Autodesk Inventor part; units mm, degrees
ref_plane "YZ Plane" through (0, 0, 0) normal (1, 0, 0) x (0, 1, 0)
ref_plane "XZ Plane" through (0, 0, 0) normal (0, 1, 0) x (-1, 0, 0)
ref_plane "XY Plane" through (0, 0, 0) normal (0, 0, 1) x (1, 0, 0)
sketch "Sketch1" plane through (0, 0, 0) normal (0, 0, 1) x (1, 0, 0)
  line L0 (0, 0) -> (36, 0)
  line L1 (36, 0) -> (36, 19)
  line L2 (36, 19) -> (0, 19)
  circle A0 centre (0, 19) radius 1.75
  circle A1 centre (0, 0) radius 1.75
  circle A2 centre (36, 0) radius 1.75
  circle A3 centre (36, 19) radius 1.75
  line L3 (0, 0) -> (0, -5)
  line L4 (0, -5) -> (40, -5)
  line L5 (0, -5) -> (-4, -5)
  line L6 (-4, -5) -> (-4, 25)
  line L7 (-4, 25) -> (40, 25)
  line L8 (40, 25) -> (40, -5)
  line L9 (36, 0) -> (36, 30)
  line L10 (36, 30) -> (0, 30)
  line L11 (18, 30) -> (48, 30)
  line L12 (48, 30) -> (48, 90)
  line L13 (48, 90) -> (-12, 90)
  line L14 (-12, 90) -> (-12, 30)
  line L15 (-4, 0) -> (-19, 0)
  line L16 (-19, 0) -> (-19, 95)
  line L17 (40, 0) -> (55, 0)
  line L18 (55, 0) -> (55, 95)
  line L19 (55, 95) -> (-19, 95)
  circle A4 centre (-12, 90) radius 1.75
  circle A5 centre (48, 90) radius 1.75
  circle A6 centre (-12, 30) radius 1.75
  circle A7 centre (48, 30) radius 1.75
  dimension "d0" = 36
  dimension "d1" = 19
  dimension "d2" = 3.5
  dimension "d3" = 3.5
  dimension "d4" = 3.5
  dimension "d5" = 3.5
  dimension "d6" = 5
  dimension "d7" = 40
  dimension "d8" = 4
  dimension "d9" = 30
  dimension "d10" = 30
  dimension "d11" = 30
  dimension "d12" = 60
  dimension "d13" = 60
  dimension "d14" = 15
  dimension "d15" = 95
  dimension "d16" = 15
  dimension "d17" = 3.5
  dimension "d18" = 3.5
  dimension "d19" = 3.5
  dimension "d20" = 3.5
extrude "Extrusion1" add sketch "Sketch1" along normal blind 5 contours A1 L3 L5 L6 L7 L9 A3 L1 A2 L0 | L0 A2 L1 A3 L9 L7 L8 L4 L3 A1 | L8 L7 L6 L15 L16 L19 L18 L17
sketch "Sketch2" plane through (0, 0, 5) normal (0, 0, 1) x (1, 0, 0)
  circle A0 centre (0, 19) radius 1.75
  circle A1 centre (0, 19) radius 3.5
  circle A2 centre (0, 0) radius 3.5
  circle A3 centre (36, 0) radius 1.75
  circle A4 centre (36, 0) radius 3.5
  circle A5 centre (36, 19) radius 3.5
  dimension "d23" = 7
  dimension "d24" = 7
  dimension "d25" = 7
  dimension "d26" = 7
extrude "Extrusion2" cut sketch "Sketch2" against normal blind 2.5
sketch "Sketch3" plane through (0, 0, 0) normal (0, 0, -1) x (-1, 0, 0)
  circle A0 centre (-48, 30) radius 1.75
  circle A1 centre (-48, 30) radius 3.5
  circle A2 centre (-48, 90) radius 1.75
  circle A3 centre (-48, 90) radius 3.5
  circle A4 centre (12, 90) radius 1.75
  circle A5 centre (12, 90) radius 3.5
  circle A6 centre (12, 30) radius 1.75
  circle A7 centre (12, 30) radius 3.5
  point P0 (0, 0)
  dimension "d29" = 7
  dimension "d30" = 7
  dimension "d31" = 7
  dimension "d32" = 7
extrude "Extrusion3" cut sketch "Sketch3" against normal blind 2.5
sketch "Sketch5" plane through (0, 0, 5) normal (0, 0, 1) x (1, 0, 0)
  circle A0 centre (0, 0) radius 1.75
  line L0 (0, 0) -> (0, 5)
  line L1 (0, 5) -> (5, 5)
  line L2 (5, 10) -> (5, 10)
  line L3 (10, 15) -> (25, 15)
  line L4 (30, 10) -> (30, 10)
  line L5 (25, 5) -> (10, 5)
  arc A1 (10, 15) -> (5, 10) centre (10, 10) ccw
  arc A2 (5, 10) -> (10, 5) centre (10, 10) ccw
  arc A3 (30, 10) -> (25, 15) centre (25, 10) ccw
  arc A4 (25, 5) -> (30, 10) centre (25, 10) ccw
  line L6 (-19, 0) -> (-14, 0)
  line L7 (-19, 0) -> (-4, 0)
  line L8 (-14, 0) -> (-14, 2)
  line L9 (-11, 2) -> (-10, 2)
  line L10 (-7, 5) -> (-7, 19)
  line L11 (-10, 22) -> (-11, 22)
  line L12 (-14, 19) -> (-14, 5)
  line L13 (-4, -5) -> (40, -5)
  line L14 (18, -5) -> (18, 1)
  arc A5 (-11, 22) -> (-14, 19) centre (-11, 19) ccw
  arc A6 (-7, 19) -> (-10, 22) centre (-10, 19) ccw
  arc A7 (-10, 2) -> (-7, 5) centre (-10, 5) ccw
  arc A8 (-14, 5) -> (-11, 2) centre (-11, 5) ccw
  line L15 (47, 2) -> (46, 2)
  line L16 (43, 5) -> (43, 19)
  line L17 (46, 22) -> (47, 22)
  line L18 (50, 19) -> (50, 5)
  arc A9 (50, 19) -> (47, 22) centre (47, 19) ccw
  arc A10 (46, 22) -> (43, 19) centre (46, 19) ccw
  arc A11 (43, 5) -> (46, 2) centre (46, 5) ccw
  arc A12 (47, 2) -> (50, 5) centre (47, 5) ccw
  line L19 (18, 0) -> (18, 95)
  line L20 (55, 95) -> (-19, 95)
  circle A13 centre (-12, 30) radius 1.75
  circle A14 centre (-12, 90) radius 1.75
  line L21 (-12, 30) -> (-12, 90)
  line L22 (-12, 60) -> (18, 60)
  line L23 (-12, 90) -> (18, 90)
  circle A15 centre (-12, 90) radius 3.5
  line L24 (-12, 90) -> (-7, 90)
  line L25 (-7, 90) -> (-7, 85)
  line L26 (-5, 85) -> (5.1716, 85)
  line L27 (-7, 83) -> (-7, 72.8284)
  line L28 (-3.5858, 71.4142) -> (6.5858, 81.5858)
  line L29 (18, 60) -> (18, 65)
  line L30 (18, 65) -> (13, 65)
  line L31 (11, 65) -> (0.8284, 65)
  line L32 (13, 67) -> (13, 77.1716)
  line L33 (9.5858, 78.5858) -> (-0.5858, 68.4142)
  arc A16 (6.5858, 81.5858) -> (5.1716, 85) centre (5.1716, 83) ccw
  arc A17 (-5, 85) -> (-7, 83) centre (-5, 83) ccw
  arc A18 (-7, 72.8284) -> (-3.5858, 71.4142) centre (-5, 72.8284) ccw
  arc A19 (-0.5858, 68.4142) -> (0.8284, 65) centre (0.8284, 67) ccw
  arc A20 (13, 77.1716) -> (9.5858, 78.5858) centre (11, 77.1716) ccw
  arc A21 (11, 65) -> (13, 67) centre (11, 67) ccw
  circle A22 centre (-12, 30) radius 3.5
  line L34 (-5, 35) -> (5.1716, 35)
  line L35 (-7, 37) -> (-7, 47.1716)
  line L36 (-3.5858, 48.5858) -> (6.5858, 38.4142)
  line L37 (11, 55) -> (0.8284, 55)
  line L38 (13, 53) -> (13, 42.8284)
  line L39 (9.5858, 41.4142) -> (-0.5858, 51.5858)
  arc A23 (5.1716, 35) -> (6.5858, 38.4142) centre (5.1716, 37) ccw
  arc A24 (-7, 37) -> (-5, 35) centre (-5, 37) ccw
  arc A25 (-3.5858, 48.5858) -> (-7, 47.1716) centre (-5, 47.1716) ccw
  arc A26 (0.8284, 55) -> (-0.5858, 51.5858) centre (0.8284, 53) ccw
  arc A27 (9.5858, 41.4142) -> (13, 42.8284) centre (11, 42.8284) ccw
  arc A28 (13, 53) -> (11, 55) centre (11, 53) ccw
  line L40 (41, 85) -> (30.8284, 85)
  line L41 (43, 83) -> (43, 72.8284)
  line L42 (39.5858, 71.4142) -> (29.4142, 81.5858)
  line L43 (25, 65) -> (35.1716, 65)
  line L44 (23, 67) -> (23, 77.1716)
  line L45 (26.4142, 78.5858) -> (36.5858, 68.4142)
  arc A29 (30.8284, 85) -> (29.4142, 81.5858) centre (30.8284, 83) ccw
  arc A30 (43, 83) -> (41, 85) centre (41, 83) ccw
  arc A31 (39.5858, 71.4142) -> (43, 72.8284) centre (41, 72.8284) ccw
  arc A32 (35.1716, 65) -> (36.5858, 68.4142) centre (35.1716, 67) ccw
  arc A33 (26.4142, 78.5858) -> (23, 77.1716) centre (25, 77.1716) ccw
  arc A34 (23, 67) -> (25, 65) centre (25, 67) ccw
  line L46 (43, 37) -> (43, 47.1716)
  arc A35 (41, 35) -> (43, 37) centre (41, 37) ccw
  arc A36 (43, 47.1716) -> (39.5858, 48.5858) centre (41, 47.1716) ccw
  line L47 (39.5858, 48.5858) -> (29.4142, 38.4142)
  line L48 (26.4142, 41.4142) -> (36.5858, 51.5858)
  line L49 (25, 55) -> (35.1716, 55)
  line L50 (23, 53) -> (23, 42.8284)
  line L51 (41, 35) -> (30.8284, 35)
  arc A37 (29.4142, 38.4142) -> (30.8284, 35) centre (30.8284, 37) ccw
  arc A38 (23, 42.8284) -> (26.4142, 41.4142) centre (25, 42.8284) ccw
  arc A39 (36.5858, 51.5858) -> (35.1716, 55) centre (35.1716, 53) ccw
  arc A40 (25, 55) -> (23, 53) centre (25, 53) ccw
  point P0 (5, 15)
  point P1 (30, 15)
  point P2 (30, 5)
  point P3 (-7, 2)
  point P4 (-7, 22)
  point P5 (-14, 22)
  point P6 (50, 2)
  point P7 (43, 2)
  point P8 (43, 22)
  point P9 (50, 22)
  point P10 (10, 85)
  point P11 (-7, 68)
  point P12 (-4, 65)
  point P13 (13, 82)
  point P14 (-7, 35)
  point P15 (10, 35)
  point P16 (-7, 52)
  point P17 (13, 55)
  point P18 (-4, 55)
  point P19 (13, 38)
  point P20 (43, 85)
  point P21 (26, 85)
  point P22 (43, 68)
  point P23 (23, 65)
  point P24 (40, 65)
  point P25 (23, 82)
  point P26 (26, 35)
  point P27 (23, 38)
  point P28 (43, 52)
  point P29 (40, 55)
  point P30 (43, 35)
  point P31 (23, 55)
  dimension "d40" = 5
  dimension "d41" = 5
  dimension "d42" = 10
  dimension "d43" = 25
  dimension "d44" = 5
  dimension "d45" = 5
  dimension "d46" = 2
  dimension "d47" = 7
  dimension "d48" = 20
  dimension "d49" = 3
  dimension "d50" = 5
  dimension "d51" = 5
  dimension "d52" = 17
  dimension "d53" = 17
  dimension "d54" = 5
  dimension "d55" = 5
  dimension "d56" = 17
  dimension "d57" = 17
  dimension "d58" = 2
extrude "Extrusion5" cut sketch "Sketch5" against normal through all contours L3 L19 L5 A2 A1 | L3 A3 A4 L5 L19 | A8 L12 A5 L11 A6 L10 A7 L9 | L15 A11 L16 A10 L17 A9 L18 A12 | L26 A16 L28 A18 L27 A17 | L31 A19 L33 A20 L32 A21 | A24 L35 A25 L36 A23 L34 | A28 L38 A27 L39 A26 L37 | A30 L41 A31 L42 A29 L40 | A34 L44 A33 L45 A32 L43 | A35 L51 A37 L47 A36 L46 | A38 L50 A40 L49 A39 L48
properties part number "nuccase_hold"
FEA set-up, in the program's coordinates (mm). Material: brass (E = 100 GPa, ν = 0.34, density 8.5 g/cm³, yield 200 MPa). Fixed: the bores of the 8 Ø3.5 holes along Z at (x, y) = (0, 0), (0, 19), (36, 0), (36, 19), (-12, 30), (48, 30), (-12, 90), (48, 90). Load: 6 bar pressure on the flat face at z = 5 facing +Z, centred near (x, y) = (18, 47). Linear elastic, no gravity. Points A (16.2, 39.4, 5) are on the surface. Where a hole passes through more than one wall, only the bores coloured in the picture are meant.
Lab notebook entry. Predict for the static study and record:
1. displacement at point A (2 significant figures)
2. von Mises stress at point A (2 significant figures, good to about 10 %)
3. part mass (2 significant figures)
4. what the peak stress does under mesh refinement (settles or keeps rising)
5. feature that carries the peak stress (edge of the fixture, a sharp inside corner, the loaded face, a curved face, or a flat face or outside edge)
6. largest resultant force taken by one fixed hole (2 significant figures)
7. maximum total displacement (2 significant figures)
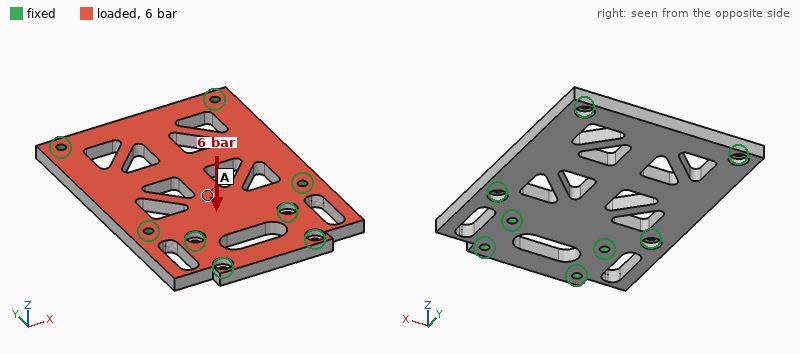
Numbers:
44 µm
17 MPa
230 g
keeps rising
edge of the fixture
770 N
75 µm
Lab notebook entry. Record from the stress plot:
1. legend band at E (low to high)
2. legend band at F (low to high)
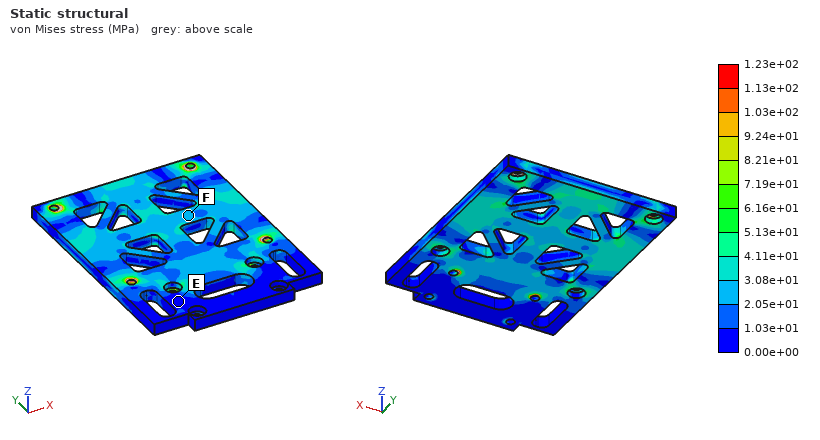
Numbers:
0.00e+00 to 1.03e+01 MPa
2.05e+01 to 3.08e+01 MPa
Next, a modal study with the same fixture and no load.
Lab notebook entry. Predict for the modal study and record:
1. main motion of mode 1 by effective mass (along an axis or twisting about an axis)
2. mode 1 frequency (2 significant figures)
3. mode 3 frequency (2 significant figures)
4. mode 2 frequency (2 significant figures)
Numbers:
along Z
2600 Hz
4100 Hz
4000 Hz
